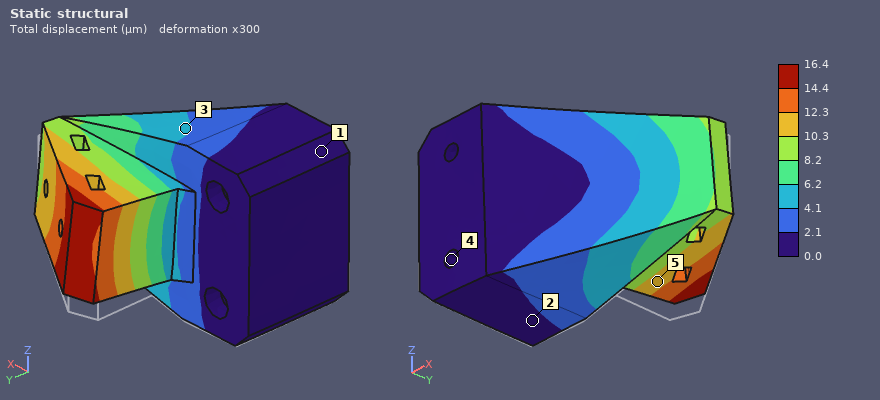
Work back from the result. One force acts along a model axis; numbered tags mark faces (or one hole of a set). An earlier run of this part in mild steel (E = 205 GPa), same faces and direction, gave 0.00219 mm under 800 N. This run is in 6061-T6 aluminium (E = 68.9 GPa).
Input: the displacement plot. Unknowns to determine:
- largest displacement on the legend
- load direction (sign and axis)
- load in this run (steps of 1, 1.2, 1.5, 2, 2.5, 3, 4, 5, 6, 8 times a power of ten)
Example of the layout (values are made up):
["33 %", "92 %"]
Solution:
["16.4 µm", "+Z", "2 kN"]
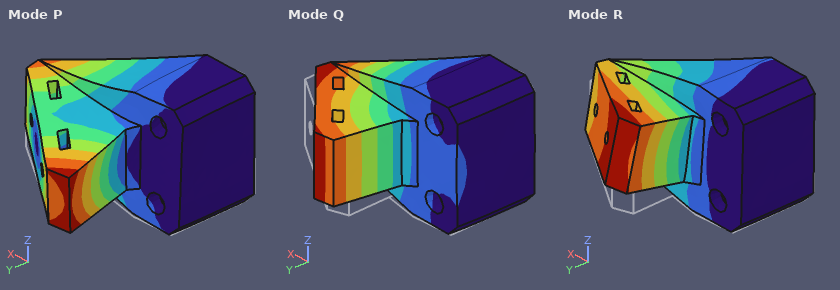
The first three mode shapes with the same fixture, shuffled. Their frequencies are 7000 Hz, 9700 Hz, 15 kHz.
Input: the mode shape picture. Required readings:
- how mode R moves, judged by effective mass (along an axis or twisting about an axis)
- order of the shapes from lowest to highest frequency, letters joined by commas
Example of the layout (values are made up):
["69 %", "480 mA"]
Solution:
["along Z", "Q, R, P"]
